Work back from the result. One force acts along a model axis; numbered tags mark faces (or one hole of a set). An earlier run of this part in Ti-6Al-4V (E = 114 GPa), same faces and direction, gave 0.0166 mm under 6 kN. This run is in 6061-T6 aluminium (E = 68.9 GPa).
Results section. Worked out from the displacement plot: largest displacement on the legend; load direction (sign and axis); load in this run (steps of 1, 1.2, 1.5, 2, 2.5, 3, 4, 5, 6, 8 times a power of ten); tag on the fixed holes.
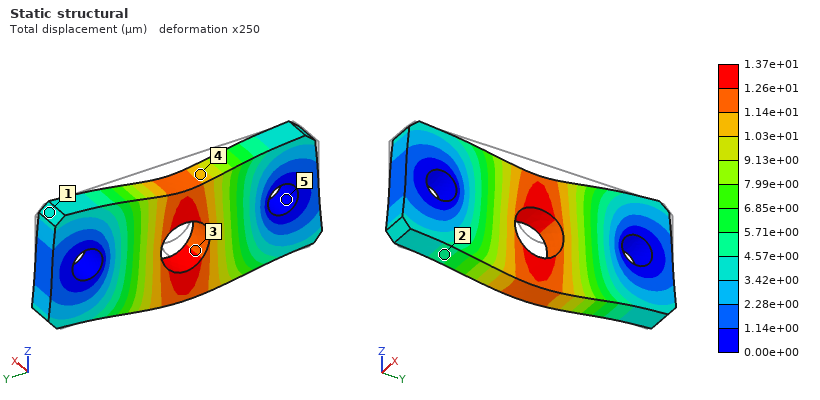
1.37e+01 µm
-Z
3 kN
5
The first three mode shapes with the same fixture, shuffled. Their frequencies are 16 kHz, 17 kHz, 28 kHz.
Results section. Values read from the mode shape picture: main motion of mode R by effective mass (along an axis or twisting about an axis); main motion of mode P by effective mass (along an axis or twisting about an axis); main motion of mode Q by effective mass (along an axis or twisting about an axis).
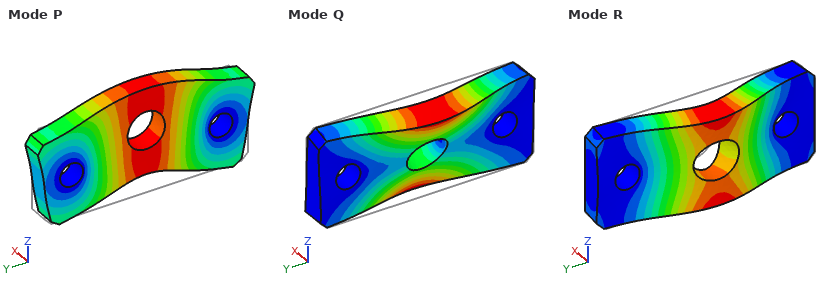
along X
along Z
twisting about Y
